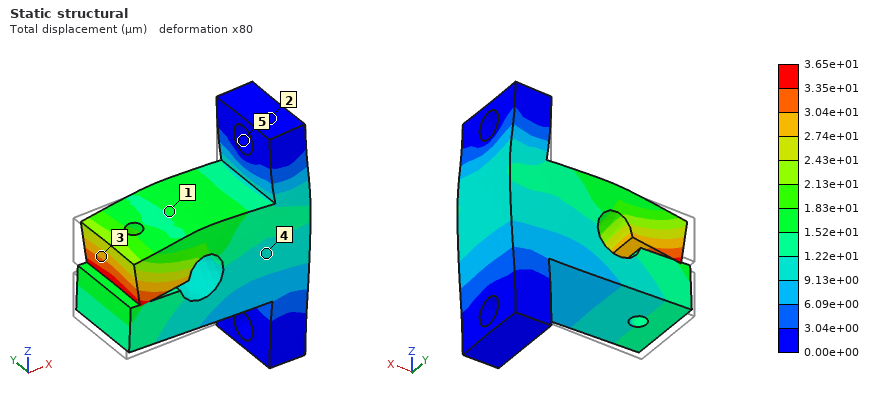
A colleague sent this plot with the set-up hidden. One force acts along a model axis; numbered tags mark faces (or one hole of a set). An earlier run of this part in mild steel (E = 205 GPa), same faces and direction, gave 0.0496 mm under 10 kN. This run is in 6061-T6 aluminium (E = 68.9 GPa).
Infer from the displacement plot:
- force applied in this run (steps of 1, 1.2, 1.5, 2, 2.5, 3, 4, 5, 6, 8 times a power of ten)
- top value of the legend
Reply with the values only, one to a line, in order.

2.5 kN
3.65e+01 µm
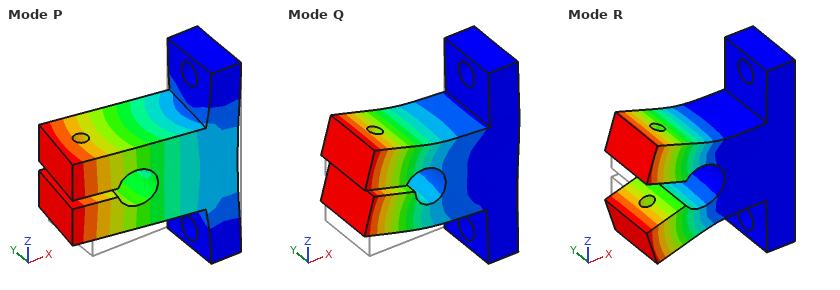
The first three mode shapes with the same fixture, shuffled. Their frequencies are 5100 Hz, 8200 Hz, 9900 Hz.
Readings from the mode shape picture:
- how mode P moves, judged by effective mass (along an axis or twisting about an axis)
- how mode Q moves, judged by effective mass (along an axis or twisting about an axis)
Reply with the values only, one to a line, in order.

along Y
along Z
